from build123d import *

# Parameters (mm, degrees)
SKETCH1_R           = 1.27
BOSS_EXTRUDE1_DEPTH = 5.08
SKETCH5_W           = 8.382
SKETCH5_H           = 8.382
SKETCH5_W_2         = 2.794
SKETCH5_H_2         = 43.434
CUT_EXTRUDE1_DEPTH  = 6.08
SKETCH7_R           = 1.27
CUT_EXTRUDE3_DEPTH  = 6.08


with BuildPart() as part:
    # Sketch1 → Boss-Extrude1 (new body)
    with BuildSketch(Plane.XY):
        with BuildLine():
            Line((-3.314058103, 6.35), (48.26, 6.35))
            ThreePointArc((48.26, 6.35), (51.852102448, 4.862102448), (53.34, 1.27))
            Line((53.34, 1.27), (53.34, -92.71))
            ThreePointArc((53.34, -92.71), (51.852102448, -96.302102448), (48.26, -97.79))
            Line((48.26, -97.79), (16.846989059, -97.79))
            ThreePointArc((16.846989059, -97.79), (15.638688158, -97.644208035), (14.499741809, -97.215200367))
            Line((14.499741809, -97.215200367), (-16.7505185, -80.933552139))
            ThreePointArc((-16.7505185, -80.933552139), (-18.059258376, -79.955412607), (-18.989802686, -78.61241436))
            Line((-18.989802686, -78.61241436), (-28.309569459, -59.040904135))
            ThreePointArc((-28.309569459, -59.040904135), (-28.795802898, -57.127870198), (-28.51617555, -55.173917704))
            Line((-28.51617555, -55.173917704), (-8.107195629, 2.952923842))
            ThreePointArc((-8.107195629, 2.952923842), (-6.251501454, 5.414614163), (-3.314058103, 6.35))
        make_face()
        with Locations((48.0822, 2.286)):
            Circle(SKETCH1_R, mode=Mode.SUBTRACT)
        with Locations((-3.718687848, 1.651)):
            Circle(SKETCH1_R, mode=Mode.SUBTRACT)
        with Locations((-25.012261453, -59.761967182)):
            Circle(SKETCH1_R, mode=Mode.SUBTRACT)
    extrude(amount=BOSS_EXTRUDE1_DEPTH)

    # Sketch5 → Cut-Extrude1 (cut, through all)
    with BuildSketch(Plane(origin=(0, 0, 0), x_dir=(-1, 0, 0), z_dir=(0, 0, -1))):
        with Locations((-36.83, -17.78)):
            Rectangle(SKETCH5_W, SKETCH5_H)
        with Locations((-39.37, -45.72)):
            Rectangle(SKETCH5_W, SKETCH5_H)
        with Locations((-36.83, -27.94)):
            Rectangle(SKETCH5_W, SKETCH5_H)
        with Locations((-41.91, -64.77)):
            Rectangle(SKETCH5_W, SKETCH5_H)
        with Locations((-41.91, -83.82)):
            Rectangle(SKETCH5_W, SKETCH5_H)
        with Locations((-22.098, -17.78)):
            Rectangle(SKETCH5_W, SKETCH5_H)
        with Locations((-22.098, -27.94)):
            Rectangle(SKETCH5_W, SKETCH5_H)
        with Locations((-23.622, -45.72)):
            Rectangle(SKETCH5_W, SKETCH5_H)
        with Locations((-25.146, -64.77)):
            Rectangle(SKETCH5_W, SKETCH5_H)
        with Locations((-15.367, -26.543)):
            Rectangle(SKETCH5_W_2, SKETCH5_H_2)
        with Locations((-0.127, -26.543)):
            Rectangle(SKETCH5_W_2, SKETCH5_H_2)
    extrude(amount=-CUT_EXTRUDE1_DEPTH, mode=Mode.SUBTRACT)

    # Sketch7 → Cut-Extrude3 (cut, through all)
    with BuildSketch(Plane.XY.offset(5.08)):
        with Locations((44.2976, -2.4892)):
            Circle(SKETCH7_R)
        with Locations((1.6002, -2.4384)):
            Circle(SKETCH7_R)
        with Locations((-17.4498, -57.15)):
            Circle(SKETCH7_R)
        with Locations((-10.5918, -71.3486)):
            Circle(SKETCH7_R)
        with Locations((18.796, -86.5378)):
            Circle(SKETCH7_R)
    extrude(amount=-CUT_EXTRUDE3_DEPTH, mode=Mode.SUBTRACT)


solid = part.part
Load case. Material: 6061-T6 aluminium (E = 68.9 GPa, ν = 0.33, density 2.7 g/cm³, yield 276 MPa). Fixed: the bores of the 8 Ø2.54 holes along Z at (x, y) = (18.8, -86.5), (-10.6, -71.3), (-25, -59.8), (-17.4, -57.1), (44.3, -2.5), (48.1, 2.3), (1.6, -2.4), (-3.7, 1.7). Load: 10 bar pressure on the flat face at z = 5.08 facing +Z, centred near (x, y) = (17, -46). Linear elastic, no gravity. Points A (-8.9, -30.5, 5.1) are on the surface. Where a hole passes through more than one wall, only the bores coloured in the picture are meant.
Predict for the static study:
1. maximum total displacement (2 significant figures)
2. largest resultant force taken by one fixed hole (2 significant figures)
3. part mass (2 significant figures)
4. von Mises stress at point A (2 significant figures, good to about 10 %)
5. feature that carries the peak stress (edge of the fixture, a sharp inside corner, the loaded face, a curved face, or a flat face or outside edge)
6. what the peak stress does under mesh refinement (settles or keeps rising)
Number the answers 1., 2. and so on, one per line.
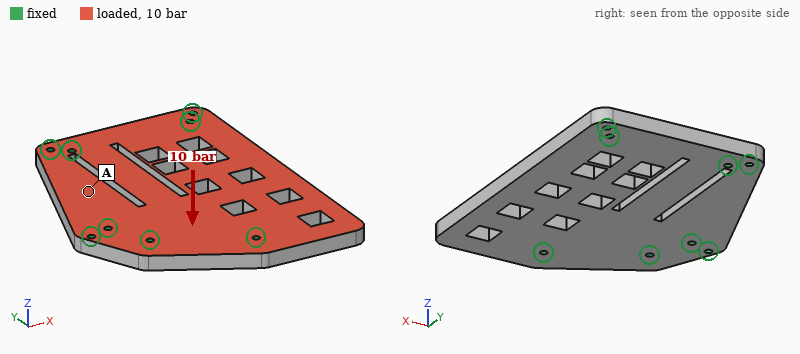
1. 0.46 mm
2. 2.2 kN
3. 87 g
4. 41 MPa
5. edge of the fixture
6. keeps rising
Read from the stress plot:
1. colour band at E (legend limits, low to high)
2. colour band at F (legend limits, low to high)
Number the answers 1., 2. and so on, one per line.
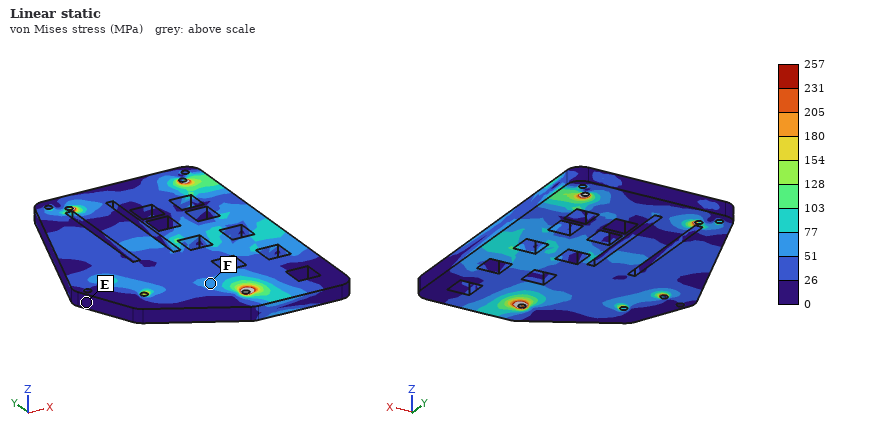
1. 0 to 26 MPa
2. 51 to 77 MPa
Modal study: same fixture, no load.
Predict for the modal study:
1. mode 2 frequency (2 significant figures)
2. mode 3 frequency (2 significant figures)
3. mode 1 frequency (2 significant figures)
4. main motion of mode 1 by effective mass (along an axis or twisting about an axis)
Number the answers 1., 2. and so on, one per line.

1. 4200 Hz
2. 5800 Hz
3. 2600 Hz
4. along Z
